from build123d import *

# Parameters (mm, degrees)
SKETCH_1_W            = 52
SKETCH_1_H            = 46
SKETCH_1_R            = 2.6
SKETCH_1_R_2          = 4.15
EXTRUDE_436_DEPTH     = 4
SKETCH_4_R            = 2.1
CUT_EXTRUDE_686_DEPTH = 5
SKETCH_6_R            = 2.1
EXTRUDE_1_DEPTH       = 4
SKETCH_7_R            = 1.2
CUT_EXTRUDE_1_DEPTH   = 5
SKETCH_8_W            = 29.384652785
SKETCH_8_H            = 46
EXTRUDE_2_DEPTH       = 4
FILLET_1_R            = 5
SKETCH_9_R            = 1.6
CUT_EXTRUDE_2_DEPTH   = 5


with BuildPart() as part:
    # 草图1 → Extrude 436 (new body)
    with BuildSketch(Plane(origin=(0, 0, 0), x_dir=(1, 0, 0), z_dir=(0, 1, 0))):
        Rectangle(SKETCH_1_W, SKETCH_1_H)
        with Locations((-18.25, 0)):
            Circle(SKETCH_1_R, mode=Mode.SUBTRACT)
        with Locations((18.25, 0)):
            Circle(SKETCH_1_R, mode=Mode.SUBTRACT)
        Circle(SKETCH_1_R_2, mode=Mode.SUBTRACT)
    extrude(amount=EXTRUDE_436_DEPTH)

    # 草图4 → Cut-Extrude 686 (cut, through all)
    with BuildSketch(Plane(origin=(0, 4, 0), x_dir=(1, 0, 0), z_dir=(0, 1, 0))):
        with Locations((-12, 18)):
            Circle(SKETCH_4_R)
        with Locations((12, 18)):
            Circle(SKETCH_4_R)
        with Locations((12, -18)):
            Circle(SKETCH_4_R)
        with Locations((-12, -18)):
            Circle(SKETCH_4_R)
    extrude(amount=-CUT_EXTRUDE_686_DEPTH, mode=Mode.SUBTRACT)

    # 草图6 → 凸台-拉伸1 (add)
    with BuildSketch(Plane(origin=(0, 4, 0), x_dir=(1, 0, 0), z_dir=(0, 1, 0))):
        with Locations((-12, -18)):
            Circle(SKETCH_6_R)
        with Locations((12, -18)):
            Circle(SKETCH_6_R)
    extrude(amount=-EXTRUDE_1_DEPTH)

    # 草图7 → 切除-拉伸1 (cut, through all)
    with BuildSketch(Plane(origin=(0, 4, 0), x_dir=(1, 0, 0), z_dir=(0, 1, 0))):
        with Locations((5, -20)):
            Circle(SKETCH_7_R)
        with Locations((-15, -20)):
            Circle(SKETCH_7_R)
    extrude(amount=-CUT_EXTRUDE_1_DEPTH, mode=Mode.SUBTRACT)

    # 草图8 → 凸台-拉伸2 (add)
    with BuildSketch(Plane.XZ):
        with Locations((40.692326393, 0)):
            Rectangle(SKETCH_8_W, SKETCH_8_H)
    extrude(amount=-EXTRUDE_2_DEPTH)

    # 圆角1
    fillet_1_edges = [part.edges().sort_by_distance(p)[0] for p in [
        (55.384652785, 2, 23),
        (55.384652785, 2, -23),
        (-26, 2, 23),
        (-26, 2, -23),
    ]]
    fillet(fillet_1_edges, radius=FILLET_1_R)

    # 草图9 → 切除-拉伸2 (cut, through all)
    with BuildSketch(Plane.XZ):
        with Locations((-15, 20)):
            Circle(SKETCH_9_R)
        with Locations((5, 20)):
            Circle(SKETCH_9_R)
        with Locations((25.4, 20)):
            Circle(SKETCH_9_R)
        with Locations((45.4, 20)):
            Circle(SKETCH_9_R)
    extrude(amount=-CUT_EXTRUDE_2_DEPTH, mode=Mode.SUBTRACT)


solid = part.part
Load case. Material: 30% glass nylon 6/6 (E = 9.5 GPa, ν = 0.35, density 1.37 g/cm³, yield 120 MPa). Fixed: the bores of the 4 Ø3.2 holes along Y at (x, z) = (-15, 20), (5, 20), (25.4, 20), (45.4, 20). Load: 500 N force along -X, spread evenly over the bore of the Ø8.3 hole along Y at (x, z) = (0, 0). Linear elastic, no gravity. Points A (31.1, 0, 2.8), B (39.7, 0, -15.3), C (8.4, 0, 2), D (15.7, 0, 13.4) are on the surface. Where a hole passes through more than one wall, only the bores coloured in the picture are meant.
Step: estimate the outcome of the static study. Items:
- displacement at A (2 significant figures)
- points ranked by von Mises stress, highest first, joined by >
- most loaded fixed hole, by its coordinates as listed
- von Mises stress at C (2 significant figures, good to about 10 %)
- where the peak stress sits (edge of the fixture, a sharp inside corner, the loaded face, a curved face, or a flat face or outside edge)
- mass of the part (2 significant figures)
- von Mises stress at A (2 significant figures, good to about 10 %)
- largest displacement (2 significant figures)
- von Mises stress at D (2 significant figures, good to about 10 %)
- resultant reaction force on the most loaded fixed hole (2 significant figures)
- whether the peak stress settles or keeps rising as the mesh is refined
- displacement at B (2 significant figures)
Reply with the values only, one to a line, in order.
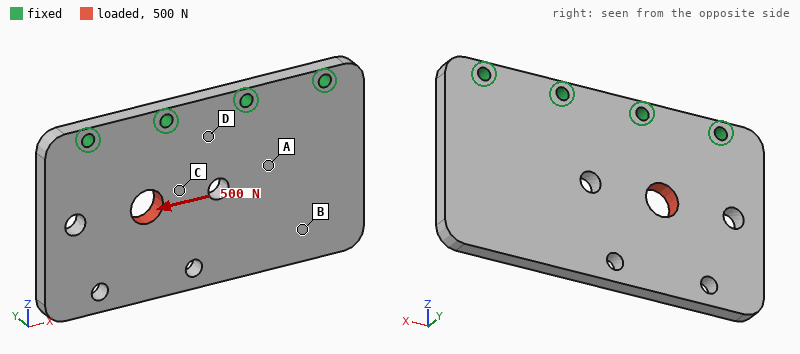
8.3 µm
C > D > A > B
(-15, 20)
5.1 MPa
edge of the fixture
20 g
2.0 MPa
21 µm
3.7 MPa
210 N
keeps rising
15 µm
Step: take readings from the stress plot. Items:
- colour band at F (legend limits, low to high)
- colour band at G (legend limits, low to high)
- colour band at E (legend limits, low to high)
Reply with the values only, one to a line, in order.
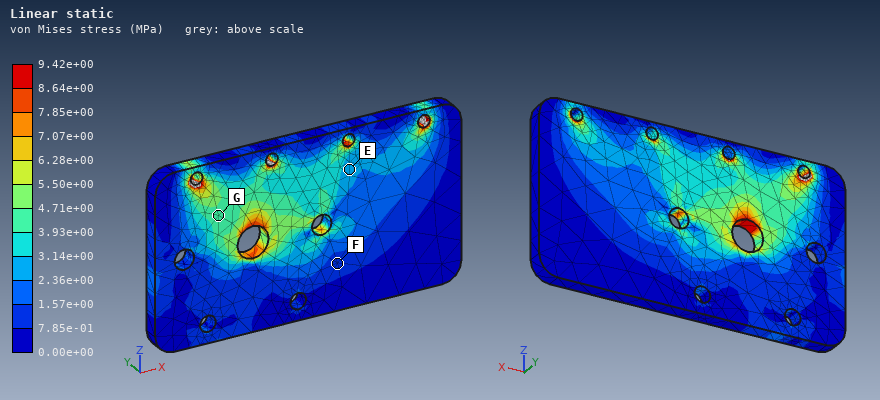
7.85e-01 to 1.57e+00 MPa
3.93e+00 to 4.71e+00 MPa
2.36e+00 to 3.14e+00 MPa
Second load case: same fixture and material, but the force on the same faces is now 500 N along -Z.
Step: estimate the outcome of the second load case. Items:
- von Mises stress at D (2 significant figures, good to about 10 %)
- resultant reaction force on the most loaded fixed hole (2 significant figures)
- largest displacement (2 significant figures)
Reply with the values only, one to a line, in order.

1.4 MPa
220 N
14 µm
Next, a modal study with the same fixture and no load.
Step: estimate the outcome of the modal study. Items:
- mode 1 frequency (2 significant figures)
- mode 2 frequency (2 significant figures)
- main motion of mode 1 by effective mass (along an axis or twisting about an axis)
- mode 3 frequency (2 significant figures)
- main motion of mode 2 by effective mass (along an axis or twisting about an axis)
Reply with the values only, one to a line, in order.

880 Hz
1400 Hz
along Y
2700 Hz
twisting about Z
